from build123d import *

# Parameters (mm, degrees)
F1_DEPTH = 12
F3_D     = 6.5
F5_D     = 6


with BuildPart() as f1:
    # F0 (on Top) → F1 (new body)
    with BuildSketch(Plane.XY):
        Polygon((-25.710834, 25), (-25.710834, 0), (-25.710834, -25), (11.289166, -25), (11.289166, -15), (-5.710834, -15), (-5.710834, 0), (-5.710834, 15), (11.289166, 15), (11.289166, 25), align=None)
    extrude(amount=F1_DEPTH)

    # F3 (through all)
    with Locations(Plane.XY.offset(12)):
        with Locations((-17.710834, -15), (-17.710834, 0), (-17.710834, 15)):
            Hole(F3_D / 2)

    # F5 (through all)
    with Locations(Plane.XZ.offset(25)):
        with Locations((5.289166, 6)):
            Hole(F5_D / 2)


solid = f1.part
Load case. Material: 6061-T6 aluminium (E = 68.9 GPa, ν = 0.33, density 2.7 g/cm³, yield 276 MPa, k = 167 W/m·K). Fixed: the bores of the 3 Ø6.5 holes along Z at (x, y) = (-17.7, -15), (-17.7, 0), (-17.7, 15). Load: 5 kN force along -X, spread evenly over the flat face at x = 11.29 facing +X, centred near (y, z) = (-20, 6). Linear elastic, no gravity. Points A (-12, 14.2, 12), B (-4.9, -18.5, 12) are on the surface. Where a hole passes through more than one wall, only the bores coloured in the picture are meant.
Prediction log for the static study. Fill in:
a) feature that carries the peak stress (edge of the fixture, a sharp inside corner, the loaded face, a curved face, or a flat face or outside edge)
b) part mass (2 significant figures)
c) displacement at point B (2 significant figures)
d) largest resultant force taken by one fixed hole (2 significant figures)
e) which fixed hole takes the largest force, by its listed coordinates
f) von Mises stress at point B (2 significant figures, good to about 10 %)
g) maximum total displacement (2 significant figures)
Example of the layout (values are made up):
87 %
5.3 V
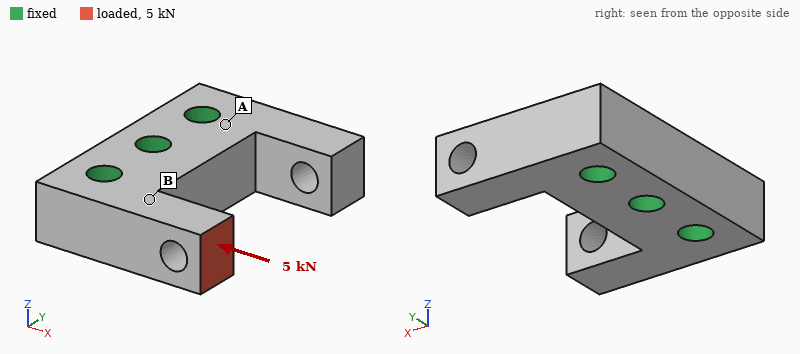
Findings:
a curved face
39 g
10 µm
5.5 kN
(-17.7, -15)
51 MPa
41 µm
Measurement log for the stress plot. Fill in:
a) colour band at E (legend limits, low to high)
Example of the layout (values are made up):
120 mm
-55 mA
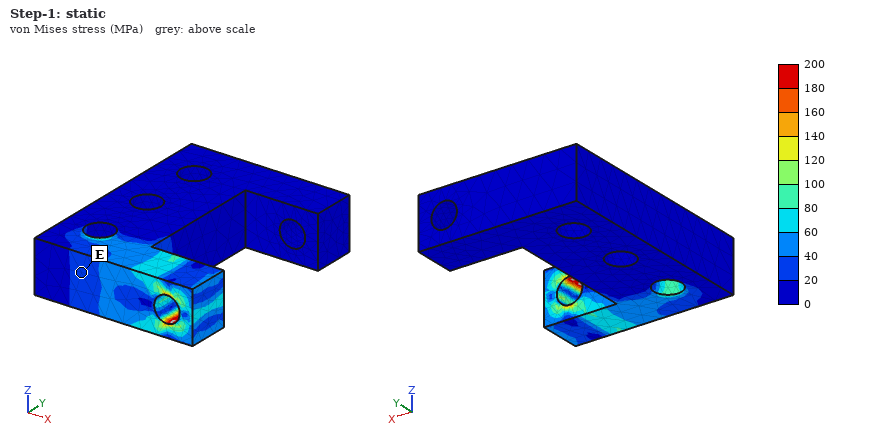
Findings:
20 to 40 MPa
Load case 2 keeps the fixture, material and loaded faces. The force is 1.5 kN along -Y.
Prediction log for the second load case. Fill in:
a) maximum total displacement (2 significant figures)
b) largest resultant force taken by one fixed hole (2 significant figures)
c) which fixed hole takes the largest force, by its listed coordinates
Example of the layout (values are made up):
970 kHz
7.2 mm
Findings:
0.12 mm
1.7 kN
(-17.7, 0)
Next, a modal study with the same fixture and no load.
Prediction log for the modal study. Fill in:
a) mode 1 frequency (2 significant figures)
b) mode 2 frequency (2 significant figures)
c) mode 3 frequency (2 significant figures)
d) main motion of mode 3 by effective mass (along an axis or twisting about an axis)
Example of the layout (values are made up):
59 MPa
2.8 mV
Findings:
13 kHz
13 kHz
15 kHz
along Y
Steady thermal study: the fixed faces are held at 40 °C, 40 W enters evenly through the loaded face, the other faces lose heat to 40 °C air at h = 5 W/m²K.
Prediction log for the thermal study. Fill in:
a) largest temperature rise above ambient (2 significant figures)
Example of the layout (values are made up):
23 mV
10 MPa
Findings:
62 K
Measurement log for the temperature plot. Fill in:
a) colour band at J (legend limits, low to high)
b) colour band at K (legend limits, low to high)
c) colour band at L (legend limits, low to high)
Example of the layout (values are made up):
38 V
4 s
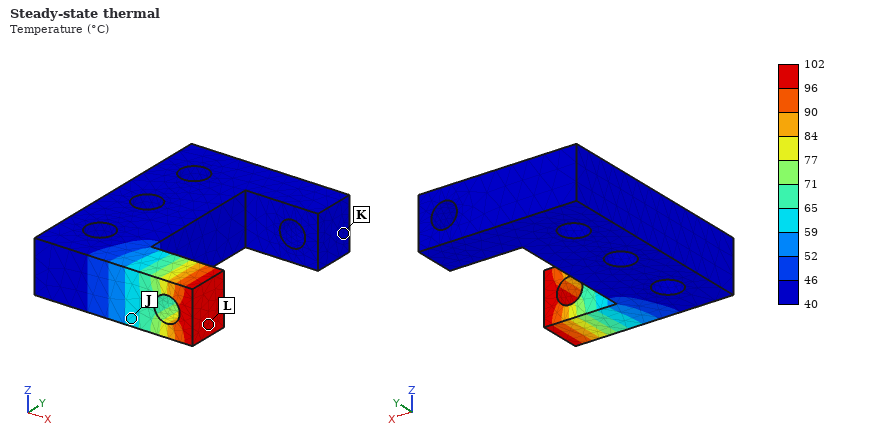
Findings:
59 to 65 °C
40 to 46 °C
96 to 102 °C
